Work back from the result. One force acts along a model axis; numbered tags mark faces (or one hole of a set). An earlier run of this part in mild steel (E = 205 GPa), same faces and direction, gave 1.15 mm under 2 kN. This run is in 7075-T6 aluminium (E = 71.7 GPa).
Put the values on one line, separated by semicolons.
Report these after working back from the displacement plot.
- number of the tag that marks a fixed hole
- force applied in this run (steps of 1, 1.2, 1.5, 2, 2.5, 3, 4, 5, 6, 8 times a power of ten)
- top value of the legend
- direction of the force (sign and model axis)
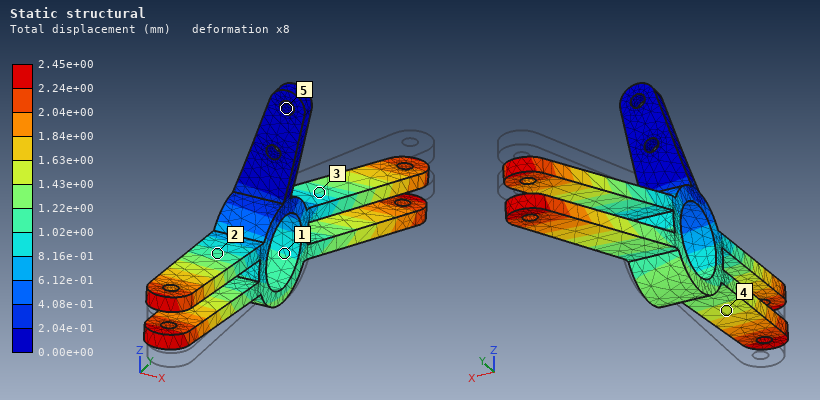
5; 1.5 kN; 2.45e+00 mm; -Y
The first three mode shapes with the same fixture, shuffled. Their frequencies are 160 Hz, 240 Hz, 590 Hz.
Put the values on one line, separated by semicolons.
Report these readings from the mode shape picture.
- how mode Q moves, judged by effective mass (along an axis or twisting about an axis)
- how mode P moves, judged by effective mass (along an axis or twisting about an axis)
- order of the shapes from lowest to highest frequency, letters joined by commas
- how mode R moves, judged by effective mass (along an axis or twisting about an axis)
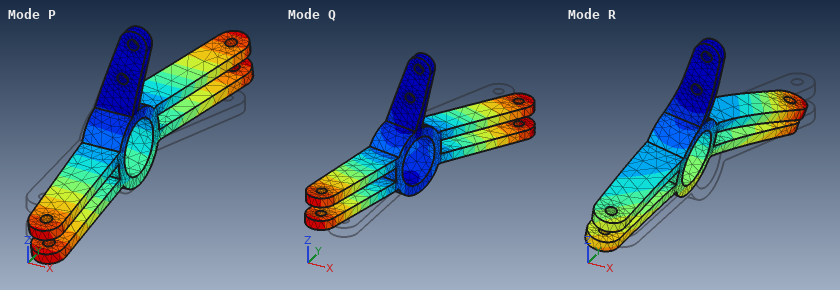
twisting about Z; along Y; P, Q, R; along X
